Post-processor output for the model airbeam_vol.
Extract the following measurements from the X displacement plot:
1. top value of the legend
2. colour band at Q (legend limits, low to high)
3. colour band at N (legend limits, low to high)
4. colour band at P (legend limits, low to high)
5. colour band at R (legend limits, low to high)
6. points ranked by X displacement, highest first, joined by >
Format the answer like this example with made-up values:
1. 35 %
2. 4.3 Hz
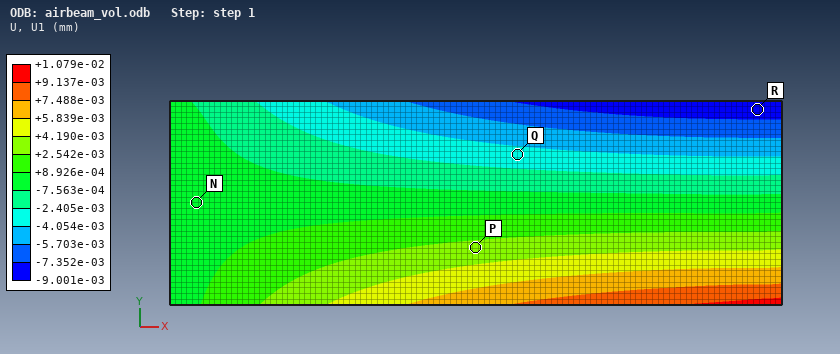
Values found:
1. +1.079e-02 mm
2. -4.054e-03 to -2.405e-03 mm
3. -7.563e-04 to +8.926e-04 mm
4. +2.542e-03 to +4.190e-03 mm
5. -9.001e-03 to -7.352e-03 mm
6. P > N > Q > R
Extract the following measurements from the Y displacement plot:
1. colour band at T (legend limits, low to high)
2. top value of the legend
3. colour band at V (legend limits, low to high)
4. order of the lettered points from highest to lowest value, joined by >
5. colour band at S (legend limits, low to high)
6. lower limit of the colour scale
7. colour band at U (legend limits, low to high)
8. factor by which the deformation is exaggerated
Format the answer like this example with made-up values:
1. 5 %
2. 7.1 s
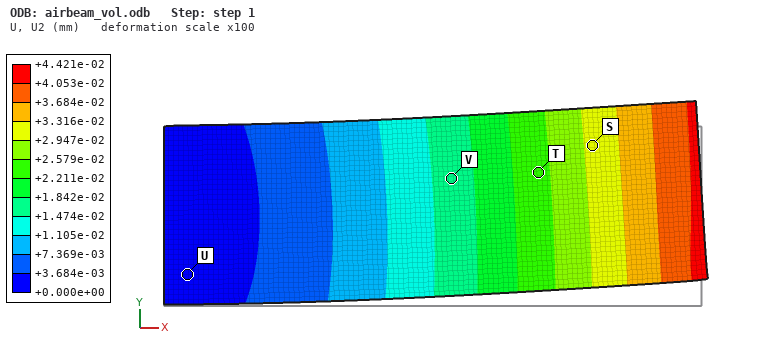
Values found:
1. +2.211e-02 to +2.579e-02 mm
2. +4.421e-02 mm
3. +1.474e-02 to +1.842e-02 mm
4. S > T > V > U
5. +2.947e-02 to +3.316e-02 mm
6. +0.000e+00 mm
7. +0.000e+00 to +3.684e-03 mm
8. 100
